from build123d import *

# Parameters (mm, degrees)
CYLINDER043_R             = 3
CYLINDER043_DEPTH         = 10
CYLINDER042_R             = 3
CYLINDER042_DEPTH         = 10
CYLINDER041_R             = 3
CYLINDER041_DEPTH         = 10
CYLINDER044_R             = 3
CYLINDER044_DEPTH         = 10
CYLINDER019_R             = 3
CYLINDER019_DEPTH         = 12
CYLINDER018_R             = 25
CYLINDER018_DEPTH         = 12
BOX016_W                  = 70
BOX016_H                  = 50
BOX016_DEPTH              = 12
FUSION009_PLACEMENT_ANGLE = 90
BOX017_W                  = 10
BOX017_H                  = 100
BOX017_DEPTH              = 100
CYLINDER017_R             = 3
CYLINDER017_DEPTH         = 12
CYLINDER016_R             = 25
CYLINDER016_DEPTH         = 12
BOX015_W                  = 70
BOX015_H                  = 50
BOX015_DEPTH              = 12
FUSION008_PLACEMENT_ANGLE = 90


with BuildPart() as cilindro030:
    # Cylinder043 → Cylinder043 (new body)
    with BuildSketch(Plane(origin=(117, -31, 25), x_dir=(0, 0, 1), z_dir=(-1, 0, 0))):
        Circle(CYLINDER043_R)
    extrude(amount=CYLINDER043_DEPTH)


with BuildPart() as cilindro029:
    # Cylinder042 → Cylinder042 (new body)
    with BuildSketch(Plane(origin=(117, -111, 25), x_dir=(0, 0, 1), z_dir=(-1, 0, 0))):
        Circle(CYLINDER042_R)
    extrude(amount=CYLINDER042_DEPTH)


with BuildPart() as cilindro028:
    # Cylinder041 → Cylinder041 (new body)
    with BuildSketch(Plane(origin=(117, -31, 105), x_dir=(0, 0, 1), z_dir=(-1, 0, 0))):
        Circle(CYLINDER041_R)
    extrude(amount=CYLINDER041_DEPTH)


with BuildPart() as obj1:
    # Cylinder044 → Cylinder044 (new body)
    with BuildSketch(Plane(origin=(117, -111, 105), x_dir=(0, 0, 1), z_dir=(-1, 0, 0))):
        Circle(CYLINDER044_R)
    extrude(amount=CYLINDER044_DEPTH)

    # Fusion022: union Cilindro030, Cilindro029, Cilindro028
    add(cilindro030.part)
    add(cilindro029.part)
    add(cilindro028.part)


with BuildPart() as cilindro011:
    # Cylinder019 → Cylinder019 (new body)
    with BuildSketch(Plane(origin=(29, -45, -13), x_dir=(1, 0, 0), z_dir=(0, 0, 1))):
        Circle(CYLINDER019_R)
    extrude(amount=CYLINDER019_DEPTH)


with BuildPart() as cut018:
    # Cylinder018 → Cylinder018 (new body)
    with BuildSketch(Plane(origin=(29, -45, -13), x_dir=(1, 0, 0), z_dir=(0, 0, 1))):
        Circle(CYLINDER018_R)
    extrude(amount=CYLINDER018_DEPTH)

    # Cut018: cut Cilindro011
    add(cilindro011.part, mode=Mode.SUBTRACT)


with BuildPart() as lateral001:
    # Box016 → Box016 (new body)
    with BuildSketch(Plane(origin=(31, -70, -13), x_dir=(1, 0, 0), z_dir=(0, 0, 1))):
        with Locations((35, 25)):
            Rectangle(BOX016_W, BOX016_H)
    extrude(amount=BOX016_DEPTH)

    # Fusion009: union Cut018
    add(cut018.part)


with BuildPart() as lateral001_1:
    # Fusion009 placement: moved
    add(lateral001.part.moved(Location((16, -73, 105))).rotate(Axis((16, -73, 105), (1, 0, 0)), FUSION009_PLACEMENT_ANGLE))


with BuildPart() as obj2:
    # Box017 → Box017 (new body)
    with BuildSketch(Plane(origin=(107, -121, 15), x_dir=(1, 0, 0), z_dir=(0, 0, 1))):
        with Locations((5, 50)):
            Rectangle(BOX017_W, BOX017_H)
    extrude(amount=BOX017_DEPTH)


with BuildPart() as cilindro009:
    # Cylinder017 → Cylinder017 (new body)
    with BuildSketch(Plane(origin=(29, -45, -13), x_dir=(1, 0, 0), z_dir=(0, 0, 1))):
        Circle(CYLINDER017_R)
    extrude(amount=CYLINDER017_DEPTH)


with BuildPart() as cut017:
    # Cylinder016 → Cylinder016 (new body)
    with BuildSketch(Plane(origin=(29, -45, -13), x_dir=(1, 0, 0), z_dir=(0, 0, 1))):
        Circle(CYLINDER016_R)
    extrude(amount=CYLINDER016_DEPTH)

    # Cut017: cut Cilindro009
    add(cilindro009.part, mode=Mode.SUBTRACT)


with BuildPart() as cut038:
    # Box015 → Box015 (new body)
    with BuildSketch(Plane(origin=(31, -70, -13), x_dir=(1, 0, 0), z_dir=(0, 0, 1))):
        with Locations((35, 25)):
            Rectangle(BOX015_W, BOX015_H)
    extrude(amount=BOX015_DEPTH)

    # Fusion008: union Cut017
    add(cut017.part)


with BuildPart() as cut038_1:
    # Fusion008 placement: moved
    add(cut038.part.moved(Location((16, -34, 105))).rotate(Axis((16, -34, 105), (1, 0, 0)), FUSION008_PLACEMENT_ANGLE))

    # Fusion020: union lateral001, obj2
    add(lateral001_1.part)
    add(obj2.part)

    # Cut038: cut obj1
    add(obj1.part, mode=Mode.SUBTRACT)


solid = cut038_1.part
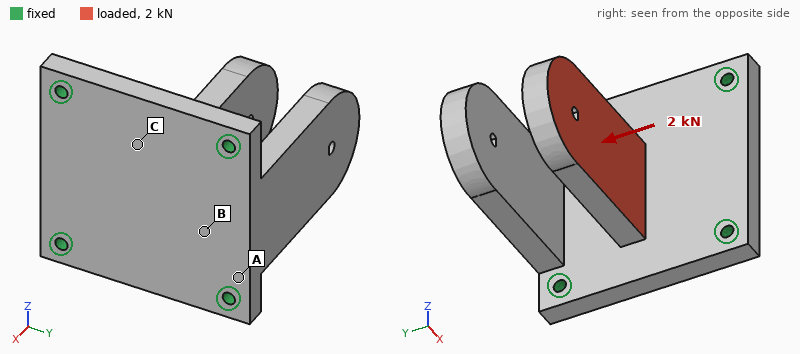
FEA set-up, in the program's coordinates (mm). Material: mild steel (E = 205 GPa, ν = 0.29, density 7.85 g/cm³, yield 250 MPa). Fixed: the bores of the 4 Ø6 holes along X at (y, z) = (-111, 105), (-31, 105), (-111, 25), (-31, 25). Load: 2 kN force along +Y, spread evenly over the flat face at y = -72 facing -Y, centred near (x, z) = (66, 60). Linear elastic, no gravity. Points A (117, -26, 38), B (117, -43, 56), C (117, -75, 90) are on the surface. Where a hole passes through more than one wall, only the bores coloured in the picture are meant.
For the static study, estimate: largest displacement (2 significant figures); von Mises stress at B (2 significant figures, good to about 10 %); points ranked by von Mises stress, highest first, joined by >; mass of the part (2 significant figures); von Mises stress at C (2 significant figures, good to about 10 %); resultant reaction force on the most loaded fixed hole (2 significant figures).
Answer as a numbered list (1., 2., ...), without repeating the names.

1. 0.15 mm
2. 10.0 MPa
3. C > B > A
4. 1.5 kg
5. 16 MPa
6. 1.0 kN
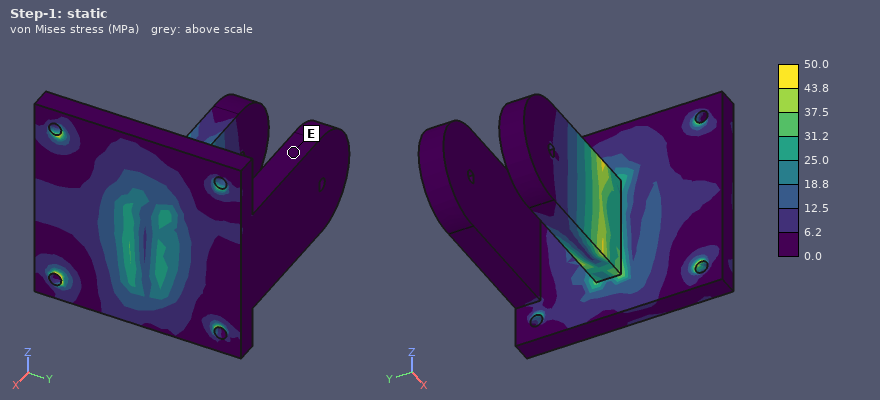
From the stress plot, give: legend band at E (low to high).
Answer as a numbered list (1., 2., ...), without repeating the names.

1. 0.0 to 6.2 MPa
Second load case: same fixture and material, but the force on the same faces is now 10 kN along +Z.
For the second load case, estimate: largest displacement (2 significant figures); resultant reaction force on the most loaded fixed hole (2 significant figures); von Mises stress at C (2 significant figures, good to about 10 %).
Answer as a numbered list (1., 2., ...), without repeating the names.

1. 0.16 mm
2. 5.0 kN
3. 68 MPa
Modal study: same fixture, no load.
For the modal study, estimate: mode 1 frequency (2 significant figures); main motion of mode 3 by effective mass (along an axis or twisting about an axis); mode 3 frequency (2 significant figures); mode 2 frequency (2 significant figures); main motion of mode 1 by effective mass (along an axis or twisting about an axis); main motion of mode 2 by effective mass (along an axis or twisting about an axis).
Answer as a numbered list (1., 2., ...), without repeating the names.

1. 1000 Hz
2. along Z
3. 2400 Hz
4. 1200 Hz
5. along Y
6. along Y
